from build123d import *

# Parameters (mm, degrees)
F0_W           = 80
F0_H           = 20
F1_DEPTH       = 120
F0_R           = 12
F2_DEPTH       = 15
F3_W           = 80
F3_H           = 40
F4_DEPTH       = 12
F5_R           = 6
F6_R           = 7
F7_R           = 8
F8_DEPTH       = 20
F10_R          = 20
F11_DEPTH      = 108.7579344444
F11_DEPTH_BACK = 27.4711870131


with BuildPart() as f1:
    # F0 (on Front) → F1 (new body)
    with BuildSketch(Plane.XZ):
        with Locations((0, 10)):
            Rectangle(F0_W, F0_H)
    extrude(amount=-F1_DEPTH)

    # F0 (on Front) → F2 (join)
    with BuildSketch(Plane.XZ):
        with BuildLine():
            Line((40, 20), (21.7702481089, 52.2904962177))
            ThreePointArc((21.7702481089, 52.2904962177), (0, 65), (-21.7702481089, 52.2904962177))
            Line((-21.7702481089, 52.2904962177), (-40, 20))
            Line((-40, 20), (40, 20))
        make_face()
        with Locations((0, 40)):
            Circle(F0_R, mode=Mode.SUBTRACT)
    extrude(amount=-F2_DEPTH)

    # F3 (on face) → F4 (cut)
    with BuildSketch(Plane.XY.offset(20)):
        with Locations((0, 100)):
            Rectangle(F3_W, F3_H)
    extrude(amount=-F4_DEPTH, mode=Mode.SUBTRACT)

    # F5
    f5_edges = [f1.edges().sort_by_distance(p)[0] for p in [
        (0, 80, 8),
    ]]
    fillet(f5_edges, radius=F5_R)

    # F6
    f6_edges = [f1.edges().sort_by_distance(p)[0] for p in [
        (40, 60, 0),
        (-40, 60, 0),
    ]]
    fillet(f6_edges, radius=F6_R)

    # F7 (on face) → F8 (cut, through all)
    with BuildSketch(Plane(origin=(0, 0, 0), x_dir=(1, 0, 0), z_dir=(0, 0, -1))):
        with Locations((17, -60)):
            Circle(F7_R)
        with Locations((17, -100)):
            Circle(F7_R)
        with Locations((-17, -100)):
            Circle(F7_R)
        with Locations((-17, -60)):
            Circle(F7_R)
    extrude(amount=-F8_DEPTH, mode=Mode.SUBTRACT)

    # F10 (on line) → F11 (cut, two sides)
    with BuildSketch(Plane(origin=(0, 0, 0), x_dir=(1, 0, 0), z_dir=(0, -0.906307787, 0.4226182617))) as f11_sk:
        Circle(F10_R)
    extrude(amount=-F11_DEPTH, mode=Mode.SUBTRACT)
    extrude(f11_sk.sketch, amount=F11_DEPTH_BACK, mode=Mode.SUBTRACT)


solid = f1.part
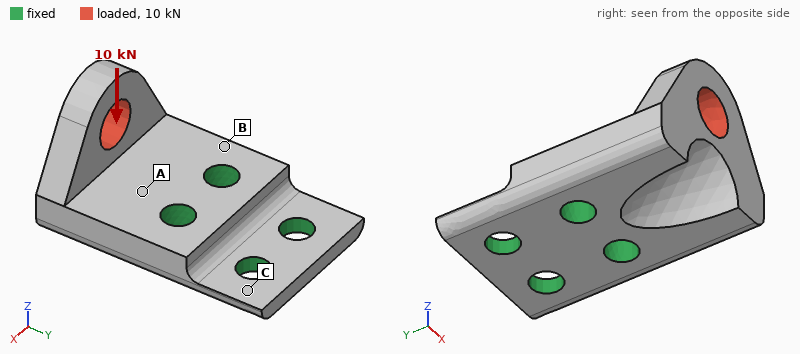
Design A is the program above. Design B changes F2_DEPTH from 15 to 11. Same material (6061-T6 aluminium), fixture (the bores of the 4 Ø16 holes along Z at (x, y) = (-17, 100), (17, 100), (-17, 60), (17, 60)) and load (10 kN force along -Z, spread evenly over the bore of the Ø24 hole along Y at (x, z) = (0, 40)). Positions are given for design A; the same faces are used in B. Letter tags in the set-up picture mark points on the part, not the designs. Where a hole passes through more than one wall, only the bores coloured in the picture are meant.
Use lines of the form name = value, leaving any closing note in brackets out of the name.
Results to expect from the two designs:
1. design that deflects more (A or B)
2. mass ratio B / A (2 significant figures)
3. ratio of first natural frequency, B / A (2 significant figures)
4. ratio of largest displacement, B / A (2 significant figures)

design that deflects more = B
mass ratio B / A = 0.95
ratio of first natural frequency, B / A = 1.0
ratio of largest displacement, B / A = 1.1
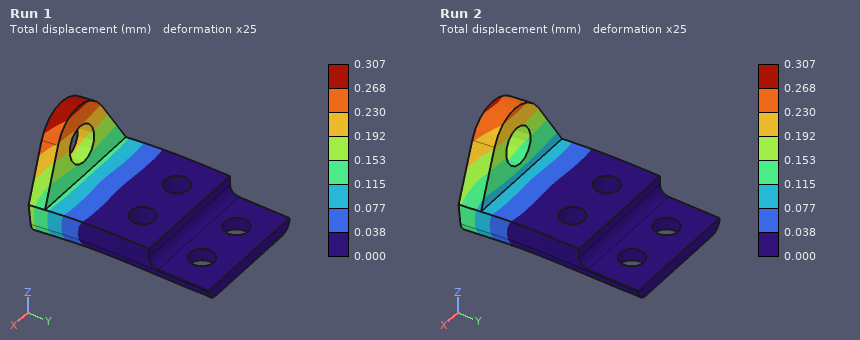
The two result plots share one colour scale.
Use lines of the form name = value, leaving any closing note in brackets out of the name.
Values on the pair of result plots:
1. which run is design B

which run is design B = Run 1
